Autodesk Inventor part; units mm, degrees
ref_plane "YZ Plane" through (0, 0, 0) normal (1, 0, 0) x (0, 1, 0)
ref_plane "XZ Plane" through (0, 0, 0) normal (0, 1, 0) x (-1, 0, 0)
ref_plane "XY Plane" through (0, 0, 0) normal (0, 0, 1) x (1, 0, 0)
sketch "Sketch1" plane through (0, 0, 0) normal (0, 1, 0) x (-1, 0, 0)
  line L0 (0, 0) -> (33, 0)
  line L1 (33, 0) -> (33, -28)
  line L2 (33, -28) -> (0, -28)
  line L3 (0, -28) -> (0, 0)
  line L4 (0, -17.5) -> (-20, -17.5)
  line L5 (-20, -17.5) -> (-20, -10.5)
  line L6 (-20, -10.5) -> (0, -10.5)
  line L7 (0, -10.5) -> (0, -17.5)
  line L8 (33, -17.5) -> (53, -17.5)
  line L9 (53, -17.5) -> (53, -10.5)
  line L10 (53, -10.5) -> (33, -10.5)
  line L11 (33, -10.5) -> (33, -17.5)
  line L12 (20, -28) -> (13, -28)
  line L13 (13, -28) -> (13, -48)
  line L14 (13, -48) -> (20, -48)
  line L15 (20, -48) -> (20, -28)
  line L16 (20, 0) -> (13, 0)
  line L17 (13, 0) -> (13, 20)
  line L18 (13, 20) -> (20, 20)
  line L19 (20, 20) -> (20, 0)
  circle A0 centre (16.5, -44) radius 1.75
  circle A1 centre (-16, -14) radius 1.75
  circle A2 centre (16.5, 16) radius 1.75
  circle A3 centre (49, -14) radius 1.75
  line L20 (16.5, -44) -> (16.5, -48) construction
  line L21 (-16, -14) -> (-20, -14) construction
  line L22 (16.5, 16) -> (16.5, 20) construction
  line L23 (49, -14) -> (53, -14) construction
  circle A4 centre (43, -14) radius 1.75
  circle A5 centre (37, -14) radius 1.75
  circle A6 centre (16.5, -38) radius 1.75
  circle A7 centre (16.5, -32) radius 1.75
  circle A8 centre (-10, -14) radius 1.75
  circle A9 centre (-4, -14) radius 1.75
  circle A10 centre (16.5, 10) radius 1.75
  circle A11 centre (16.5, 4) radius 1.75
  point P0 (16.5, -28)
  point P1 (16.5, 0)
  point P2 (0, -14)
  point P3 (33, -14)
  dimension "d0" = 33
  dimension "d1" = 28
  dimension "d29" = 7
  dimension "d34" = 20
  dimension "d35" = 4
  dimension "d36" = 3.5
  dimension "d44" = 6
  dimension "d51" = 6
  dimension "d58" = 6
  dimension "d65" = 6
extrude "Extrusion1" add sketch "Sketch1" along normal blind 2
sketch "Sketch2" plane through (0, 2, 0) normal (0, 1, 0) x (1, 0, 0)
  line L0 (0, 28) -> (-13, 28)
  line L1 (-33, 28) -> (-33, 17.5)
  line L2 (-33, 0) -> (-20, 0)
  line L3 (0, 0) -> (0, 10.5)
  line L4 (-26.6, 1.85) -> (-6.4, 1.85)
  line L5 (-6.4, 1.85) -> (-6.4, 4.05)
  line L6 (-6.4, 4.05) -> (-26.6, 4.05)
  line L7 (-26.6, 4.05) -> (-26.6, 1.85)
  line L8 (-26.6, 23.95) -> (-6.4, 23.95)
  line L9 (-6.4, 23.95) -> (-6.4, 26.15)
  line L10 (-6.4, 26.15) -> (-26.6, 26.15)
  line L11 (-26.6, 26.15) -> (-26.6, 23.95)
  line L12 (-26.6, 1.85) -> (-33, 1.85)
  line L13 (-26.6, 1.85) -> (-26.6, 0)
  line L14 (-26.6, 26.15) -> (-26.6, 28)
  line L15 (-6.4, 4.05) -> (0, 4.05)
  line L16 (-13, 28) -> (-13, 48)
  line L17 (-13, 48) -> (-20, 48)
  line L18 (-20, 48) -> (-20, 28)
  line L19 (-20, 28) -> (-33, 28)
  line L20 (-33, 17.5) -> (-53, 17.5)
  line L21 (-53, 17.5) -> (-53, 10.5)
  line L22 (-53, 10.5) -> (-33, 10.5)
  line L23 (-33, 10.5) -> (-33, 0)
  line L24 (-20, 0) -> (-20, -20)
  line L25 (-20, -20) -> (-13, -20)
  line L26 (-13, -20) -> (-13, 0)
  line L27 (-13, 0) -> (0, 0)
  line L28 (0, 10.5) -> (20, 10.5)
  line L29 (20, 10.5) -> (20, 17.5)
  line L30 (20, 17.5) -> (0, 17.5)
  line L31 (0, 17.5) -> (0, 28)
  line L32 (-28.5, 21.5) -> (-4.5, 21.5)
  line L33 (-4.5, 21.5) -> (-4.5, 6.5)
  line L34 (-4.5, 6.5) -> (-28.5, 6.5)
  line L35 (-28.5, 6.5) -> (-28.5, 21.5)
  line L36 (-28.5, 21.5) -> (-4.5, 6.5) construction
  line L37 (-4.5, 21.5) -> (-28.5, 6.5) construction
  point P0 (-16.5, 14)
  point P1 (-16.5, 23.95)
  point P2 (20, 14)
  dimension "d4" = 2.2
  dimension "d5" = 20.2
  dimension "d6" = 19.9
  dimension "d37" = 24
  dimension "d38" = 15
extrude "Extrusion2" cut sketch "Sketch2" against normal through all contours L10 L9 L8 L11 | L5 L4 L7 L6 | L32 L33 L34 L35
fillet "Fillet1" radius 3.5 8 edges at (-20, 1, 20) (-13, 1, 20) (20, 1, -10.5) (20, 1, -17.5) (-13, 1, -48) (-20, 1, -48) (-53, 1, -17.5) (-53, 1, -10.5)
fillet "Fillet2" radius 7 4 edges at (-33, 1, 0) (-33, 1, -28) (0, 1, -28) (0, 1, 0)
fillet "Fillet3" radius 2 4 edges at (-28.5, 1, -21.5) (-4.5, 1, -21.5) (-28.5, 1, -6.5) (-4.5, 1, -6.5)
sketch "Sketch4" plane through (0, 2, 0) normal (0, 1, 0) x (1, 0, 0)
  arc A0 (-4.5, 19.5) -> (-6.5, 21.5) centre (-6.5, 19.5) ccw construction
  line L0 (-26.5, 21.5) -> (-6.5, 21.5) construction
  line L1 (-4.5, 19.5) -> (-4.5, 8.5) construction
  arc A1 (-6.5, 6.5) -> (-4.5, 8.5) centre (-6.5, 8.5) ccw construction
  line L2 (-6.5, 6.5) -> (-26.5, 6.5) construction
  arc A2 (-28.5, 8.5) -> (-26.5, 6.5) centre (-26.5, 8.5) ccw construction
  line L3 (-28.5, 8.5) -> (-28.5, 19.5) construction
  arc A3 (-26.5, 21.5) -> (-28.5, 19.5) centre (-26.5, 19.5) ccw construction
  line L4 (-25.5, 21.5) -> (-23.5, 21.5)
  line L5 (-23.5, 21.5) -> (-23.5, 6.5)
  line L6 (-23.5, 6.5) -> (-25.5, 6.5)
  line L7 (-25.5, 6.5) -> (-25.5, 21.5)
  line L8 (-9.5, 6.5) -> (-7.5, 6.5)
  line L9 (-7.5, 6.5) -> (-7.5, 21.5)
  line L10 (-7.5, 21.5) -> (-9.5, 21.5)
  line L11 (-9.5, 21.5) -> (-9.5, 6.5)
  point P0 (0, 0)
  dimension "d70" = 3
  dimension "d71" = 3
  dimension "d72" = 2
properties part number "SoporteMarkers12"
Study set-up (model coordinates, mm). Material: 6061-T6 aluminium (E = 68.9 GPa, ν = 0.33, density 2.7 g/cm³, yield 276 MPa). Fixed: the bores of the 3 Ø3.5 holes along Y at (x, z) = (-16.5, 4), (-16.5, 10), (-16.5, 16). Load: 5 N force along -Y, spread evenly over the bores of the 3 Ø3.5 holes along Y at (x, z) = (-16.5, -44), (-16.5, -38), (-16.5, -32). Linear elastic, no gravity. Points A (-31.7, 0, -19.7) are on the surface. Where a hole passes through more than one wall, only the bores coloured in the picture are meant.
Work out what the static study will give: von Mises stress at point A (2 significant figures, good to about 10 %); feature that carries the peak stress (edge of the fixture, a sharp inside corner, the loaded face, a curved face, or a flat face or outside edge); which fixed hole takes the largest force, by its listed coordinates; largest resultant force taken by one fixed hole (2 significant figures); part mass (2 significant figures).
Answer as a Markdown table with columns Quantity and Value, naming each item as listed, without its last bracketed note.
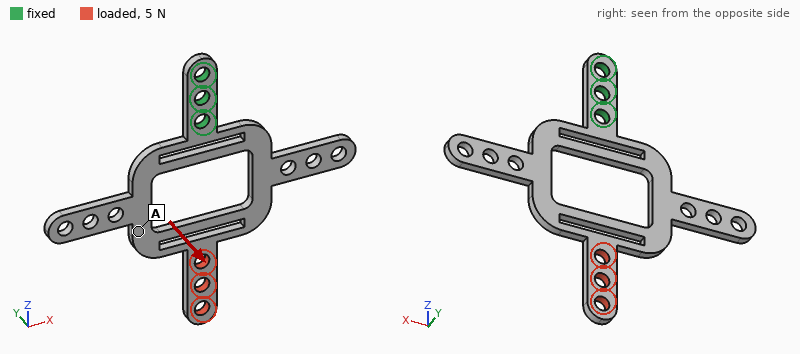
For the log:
| Quantity | Value |
|---|---|
| von Mises stress at point A | 15 MPa |
| feature that carries the peak stress | a flat face or outside edge |
| which fixed hole takes the largest force, by its listed coordinates | (-16.5, 4) |
| largest resultant force taken by one fixed hole | 6.0 N |
| part mass | 4.6 g |
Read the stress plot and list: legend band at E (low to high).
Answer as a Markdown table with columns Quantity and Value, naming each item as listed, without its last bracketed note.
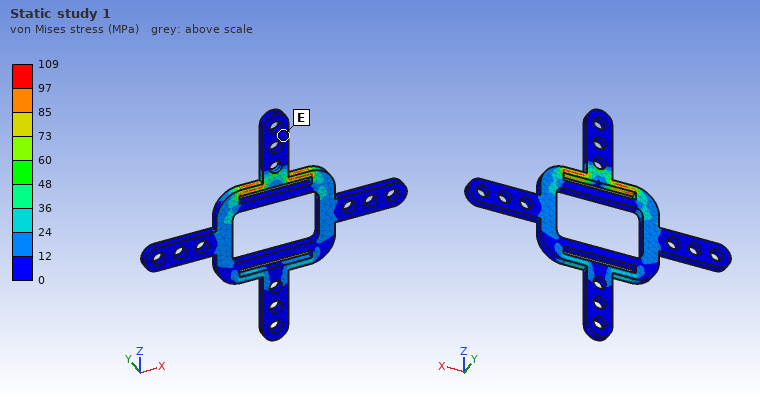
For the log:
| Quantity | Value |
|---|---|
| legend band at E | 0 to 12 MPa |
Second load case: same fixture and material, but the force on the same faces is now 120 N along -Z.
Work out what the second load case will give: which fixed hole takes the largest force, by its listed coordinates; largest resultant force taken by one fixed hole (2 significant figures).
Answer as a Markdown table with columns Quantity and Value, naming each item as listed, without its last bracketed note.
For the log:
| Quantity | Value |
|---|---|
| which fixed hole takes the largest force, by its listed coordinates | (-16.5, 4) |
| largest resultant force taken by one fixed hole | 110 N |
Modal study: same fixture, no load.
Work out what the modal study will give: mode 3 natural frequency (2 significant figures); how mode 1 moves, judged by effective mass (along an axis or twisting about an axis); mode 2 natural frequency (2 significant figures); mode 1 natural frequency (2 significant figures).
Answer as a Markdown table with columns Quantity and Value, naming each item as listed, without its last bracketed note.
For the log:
| Quantity | Value |
|---|---|
| mode 3 natural frequency | 780 Hz |
| how mode 1 moves, judged by effective mass | along Y |
| mode 2 natural frequency | 760 Hz |
| mode 1 natural frequency | 370 Hz |
